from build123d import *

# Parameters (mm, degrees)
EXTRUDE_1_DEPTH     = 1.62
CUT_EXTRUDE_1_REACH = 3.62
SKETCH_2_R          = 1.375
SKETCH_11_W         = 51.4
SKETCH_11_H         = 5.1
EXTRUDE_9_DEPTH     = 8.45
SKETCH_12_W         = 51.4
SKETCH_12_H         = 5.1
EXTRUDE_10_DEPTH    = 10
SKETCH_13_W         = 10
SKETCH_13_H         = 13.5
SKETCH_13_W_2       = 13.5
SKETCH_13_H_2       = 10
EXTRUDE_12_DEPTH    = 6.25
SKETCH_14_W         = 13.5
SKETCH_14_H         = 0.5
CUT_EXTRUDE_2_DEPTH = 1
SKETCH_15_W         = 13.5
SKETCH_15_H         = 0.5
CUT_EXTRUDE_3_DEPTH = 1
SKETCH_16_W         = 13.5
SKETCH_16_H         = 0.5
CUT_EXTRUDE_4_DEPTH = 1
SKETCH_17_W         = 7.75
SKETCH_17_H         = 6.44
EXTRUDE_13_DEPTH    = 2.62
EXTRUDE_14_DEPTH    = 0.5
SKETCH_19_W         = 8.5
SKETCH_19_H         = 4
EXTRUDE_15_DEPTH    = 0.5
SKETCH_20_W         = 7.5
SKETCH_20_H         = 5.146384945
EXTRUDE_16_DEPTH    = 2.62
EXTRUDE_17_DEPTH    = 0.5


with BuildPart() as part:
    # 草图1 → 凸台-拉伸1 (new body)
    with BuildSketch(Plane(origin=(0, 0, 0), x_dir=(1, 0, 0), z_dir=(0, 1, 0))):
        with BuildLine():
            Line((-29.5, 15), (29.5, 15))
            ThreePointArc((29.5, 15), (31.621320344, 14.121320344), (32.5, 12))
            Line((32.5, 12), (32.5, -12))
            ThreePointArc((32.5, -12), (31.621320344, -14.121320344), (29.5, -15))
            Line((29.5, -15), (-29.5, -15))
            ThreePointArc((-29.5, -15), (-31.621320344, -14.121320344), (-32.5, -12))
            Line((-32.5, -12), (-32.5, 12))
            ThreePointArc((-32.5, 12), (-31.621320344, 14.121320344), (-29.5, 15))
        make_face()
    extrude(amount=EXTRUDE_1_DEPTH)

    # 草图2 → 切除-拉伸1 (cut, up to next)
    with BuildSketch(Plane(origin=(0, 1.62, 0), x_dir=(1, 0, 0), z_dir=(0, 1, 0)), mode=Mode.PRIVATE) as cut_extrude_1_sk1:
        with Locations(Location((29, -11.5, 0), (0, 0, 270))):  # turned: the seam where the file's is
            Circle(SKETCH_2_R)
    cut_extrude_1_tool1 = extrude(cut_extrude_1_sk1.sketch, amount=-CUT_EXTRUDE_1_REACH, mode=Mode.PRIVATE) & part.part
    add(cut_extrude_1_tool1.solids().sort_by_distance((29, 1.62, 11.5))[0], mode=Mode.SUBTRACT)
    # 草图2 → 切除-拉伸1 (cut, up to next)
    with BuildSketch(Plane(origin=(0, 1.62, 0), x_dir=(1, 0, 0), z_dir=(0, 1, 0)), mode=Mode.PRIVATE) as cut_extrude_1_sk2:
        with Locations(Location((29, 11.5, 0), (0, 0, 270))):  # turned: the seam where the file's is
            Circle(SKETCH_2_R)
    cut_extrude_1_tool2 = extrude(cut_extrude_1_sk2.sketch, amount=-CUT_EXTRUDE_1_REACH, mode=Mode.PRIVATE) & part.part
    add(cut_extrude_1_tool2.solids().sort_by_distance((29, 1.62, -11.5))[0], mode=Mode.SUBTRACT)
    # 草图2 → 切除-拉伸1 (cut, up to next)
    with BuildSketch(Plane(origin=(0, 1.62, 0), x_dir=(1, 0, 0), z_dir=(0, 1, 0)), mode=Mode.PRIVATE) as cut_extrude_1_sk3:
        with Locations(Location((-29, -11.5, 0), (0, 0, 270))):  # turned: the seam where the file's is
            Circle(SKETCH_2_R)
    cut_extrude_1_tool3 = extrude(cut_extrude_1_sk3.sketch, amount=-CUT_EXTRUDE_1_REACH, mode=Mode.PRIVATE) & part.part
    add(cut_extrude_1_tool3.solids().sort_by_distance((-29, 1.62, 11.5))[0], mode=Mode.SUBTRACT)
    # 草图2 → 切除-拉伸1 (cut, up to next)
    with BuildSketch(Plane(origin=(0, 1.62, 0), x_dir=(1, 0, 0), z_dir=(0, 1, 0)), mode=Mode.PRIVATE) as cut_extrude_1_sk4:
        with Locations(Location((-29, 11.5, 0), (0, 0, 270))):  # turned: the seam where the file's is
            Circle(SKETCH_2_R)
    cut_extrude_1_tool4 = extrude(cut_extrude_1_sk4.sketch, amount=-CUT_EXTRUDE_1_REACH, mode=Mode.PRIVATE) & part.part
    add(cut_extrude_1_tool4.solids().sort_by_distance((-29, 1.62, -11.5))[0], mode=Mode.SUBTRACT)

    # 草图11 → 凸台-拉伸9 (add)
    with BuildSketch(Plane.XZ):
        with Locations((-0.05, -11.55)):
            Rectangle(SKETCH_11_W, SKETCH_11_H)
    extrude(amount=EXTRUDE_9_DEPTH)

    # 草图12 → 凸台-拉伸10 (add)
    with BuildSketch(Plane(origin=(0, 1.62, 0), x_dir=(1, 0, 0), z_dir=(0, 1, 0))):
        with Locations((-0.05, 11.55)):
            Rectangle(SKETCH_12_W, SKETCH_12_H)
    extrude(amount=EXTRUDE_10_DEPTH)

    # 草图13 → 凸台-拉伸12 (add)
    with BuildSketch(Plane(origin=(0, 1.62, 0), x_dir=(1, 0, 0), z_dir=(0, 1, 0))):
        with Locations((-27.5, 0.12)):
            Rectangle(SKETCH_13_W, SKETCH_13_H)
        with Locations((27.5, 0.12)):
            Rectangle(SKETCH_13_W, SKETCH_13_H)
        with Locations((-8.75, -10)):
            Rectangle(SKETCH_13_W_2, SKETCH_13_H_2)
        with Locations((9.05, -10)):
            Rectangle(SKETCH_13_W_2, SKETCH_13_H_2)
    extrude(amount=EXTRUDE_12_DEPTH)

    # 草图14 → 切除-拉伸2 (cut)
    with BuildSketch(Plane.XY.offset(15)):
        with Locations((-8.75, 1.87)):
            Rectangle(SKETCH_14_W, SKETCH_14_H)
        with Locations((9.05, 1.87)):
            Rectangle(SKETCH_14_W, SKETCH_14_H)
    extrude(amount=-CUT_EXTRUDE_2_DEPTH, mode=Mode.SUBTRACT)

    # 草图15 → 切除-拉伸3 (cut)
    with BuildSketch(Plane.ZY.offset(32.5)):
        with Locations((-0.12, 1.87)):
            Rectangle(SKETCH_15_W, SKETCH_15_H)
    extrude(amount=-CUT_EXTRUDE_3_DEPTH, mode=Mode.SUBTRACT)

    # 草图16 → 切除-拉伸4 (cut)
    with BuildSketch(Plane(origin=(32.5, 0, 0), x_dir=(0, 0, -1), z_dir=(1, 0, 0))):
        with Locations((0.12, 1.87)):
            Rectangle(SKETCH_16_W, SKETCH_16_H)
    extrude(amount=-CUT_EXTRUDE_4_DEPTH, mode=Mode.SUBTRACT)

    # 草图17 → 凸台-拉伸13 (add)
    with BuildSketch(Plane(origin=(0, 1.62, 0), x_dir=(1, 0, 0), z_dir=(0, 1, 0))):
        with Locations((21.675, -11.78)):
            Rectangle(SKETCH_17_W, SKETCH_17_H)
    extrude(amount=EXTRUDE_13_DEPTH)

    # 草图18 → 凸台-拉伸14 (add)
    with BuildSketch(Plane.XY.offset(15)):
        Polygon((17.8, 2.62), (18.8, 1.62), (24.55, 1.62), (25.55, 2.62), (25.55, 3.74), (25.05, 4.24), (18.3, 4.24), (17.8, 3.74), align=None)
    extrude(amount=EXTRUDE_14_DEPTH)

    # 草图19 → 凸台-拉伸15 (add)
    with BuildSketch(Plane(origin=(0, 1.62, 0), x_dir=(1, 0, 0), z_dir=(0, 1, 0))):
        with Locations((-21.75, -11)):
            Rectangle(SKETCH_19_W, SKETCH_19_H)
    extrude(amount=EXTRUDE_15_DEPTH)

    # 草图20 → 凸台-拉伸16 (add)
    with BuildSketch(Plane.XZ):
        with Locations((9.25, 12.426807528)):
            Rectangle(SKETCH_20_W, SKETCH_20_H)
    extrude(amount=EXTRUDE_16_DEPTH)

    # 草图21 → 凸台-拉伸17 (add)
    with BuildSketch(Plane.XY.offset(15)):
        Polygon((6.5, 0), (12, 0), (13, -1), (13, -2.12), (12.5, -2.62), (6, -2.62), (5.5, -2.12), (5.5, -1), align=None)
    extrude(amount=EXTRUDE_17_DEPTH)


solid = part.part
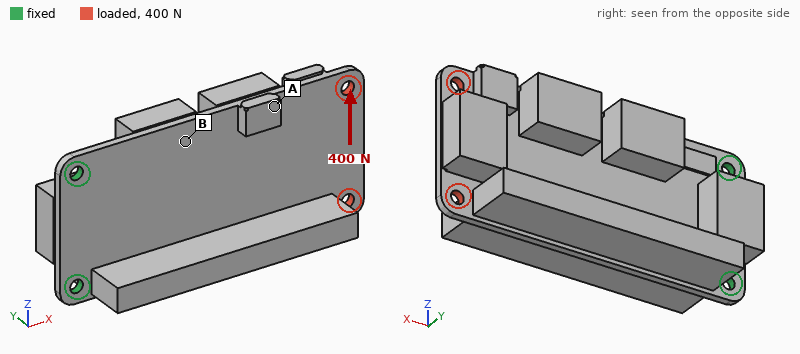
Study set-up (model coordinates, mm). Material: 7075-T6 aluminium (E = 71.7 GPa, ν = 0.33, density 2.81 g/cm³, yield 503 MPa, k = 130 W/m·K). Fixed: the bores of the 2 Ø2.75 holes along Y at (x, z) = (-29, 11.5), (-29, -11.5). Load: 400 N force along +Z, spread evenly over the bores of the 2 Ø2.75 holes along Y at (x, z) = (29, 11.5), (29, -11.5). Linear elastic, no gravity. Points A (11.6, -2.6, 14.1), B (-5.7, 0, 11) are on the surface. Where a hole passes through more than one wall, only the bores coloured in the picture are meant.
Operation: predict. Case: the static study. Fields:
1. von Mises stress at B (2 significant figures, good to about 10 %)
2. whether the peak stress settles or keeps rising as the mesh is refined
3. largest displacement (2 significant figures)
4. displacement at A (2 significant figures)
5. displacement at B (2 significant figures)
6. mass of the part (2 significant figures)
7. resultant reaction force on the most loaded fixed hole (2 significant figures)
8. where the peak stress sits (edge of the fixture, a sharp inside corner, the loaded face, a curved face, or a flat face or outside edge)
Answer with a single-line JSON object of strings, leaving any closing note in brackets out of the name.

{"von Mises stress at B": "27 MPa", "whether the peak stress settles or keeps rising as the mesh is refined": "keeps rising", "largest displacement": "88 µm", "displacement at A": "57 µm", "displacement at B": "28 µm", "mass of the part": "32 g", "resultant reaction force on the most loaded fixed hole": "1.0 kN", "where the peak stress sits": "edge of the fixture"}
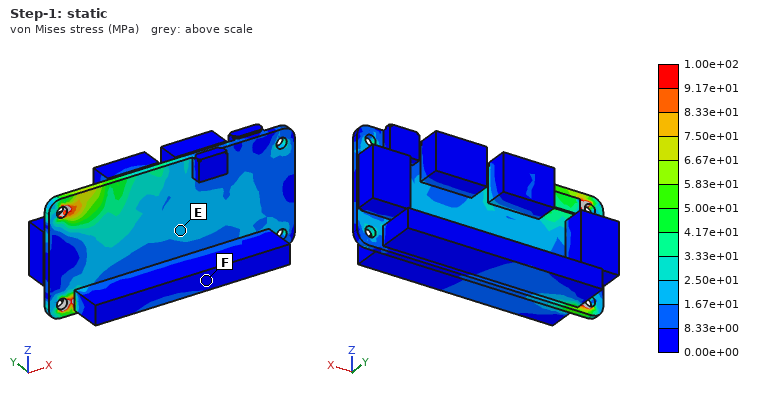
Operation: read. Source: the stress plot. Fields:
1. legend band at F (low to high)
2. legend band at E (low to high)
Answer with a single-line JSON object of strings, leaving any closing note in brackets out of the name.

{"legend band at F": "0.00e+00 to 8.33e+00 MPa", "legend band at E": "1.67e+01 to 2.50e+01 MPa"}
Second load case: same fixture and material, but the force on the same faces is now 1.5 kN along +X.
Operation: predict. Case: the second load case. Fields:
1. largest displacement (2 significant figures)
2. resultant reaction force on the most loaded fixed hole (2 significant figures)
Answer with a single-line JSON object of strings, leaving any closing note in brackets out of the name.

{"largest displacement": "49 µm", "resultant reaction force on the most loaded fixed hole": "760 N"}
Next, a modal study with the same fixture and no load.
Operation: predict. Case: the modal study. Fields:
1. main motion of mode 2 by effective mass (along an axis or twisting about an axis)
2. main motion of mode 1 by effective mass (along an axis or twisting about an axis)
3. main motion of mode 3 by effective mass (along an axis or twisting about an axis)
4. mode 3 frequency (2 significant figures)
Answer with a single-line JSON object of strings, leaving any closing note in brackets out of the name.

{"main motion of mode 2 by effective mass": "twisting about X", "main motion of mode 1 by effective mass": "along Y", "main motion of mode 3 by effective mass": "along Z", "mode 3 frequency": "3500 Hz"}
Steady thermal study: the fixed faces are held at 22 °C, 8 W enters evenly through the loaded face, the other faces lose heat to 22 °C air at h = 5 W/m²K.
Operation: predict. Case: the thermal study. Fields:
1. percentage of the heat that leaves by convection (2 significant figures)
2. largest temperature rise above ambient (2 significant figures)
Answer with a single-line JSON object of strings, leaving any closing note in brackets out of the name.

{"percentage of the heat that leaves by convection": "8.7 %", "largest temperature rise above ambient": "43 K"}
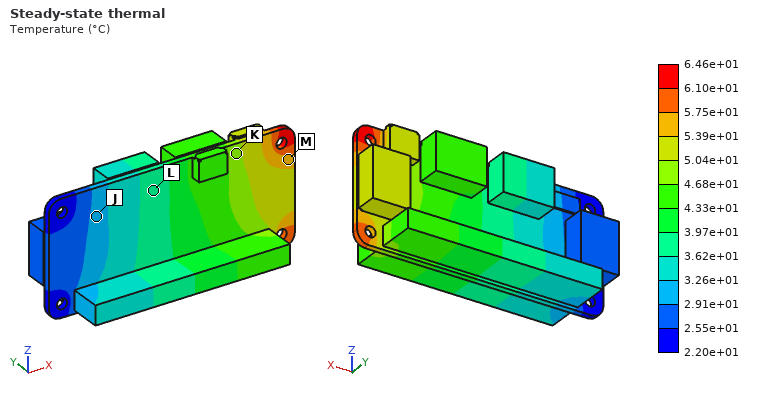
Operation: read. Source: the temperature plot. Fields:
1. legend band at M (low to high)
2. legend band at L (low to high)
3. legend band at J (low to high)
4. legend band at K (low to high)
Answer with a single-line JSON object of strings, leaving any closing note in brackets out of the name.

{"legend band at M": "5.39e+01 to 5.75e+01 °C", "legend band at L": "3.62e+01 to 3.97e+01 °C", "legend band at J": "2.91e+01 to 3.26e+01 °C", "legend band at K": "4.68e+01 to 5.04e+01 °C"}
